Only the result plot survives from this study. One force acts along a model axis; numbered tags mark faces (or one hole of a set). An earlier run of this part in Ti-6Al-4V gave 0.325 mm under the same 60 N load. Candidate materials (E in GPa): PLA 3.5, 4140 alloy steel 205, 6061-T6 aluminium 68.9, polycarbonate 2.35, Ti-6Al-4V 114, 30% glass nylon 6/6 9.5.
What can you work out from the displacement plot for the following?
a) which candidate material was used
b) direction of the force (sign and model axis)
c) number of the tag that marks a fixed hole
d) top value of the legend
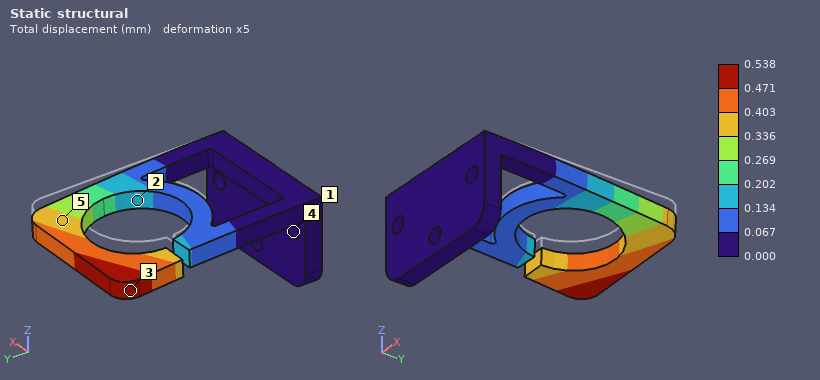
6061-T6 aluminium
-Z
4
0.538 mm
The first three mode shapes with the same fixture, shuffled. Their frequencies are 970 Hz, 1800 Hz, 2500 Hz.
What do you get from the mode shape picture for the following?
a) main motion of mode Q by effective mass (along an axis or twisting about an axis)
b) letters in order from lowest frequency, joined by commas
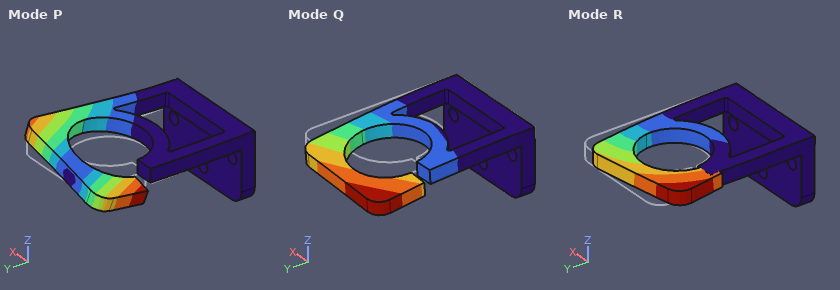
along Z
Q, R, P
